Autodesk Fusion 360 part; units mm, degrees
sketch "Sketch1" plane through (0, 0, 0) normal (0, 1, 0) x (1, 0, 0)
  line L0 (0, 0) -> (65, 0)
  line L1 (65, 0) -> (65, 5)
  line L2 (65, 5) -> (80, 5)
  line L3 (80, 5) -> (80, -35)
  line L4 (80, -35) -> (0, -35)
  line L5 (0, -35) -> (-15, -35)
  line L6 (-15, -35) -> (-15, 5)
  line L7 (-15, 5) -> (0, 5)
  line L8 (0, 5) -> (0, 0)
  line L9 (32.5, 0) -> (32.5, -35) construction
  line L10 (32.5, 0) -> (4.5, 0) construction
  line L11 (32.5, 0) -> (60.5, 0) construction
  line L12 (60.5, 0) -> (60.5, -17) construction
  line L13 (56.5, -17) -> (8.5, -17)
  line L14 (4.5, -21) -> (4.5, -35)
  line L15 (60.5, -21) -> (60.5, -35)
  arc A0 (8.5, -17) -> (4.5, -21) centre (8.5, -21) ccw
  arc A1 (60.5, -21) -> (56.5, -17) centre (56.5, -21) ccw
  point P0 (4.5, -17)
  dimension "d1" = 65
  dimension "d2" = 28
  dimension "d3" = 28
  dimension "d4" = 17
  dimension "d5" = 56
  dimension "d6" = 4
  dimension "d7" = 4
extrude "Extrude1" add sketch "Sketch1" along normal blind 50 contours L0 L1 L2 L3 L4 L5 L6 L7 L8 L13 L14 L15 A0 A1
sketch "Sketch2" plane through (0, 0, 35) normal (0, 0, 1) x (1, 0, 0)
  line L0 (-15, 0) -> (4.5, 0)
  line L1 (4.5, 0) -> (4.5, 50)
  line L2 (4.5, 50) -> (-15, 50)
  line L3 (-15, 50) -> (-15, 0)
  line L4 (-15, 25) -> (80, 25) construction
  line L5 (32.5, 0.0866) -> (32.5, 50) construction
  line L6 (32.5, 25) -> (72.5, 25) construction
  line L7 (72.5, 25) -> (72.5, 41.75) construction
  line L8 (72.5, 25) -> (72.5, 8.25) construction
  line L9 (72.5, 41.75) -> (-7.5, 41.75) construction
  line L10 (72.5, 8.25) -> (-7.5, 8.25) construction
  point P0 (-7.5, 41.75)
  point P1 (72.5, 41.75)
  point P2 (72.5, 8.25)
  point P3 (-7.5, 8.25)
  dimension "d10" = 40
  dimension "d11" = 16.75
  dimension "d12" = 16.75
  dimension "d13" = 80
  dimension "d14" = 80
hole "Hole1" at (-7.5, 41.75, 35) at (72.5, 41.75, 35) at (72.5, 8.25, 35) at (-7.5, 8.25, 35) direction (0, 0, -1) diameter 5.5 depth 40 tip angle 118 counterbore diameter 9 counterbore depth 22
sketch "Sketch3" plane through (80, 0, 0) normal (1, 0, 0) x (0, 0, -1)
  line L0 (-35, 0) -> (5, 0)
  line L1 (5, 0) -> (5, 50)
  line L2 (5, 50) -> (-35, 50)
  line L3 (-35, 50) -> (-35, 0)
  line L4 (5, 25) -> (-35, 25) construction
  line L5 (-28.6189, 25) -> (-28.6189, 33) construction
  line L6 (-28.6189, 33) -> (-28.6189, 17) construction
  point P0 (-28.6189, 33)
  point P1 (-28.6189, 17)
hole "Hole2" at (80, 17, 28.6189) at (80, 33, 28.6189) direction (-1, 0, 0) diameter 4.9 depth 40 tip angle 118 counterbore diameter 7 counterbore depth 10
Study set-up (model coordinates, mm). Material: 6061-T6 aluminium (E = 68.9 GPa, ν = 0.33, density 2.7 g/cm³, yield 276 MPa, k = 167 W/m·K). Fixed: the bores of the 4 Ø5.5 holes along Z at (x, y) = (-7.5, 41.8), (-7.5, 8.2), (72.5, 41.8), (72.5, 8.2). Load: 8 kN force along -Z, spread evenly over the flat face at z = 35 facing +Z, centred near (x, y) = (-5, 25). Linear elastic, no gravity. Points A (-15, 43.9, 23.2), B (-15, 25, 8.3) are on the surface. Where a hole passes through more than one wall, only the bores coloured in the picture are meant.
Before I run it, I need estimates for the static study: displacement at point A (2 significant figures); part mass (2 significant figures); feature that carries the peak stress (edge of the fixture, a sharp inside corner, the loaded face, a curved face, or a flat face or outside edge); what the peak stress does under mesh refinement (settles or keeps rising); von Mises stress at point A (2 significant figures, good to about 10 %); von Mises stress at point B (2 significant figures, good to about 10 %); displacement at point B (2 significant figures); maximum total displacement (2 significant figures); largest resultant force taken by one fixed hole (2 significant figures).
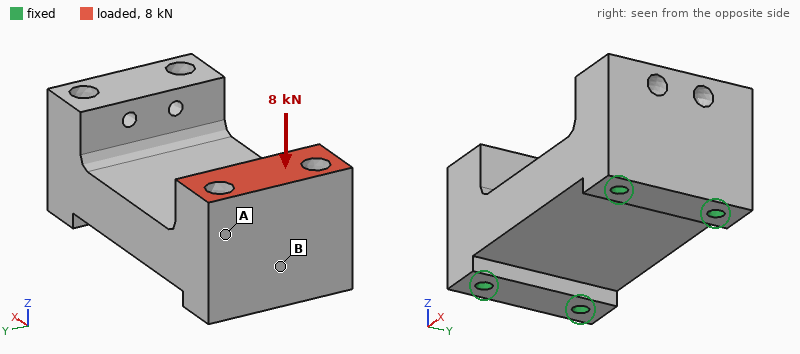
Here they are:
3.3 µm
310 g
edge of the fixture
keeps rising
11 MPa
3.7 MPa
2.7 µm
5.8 µm
4.0 kN
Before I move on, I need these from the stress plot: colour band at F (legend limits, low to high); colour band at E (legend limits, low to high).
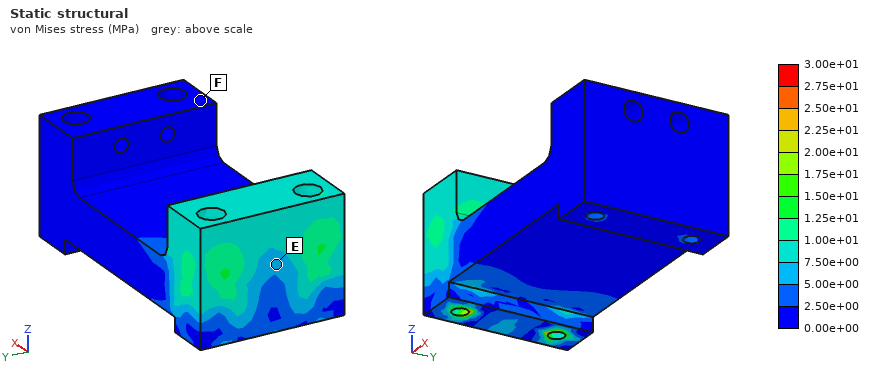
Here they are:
0.00e+00 to 2.50e+00 MPa
5.00e+00 to 7.50e+00 MPa
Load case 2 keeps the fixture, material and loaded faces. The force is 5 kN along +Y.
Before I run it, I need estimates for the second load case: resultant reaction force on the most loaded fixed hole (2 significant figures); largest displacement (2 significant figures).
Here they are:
4.2 kN
17 µm
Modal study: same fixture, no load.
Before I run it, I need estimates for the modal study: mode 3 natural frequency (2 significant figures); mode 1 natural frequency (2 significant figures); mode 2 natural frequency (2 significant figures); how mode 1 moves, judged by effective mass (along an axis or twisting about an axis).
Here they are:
15 kHz
9100 Hz
14 kHz
along Z
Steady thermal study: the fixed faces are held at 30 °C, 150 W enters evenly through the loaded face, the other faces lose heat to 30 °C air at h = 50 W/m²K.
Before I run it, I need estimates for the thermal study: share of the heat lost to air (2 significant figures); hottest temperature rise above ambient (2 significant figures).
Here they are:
4.0 %
31 K
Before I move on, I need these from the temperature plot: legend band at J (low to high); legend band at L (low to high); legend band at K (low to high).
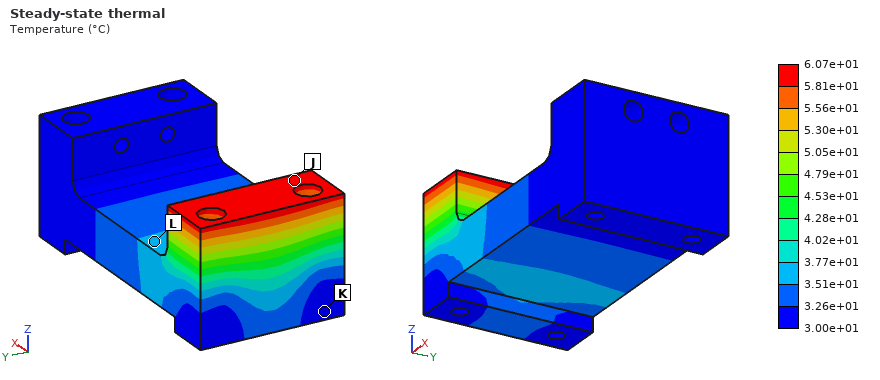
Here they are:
5.81e+01 to 6.07e+01 °C
3.51e+01 to 3.77e+01 °C
3.00e+01 to 3.26e+01 °C
